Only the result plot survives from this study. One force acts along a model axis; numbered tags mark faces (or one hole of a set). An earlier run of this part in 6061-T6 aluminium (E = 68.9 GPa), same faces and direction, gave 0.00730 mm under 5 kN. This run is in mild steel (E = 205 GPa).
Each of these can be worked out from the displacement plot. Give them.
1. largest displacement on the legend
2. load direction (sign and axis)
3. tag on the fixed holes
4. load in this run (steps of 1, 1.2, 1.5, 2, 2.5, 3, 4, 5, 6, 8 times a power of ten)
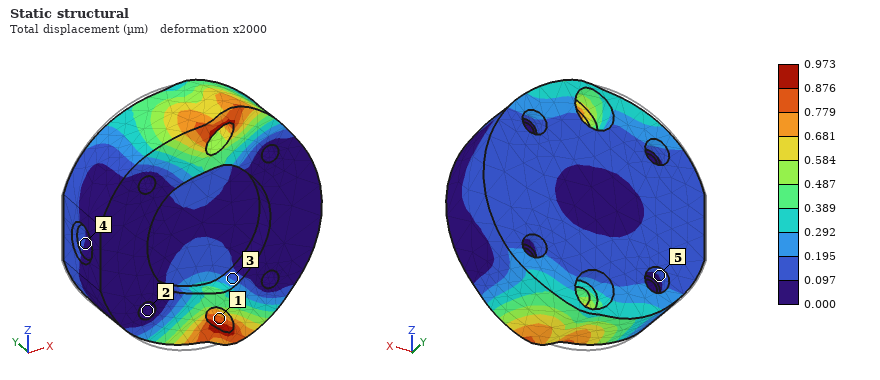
0.973 µm
+X
2
2 kN
